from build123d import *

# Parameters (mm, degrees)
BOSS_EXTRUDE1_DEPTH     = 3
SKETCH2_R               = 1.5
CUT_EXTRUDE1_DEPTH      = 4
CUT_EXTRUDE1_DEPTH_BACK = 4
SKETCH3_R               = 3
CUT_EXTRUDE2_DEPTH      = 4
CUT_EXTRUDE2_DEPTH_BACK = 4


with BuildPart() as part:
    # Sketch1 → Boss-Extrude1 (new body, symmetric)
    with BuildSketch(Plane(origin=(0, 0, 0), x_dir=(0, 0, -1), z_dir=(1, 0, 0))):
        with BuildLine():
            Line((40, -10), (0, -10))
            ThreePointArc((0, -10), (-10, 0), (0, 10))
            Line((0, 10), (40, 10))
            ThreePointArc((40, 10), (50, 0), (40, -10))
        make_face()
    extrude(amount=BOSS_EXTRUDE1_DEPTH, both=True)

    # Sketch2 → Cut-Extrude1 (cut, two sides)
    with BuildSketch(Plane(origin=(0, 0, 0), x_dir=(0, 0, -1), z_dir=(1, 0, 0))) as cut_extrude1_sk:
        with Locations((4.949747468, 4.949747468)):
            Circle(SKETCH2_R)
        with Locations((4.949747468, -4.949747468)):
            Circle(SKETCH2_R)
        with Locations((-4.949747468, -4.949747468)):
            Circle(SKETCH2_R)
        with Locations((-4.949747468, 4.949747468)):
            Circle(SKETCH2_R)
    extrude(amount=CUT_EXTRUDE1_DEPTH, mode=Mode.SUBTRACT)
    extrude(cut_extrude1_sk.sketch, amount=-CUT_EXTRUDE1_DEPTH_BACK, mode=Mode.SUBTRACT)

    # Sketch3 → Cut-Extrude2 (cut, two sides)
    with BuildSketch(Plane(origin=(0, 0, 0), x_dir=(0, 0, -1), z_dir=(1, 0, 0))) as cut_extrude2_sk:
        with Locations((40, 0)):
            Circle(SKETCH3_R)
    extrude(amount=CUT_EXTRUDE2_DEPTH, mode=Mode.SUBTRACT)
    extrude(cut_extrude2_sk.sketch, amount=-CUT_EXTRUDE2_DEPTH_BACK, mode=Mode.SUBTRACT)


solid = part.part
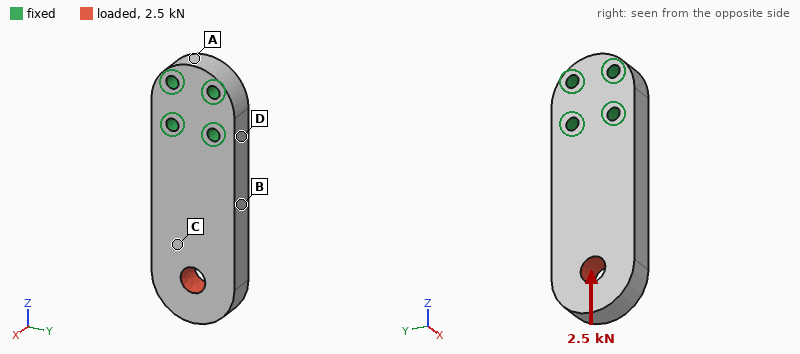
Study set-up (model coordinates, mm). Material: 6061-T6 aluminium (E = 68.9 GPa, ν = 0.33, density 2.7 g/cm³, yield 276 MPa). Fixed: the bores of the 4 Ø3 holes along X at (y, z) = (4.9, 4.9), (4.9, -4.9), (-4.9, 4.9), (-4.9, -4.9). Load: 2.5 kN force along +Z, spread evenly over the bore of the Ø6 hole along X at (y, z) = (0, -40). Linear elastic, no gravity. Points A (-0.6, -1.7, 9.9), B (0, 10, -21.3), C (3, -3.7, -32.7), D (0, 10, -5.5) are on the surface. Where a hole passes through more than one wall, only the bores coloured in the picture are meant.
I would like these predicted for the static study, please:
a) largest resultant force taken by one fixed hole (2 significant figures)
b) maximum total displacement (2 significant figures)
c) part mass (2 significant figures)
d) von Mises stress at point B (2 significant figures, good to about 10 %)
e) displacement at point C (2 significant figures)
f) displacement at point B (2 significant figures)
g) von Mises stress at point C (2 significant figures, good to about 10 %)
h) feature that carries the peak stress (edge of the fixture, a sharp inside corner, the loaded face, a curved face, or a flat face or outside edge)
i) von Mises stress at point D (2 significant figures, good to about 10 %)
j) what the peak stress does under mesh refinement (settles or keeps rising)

1.1 kN
14 µm
17 g
21 MPa
8.6 µm
5.2 µm
25 MPa
edge of the fixture
13 MPa
keeps rising
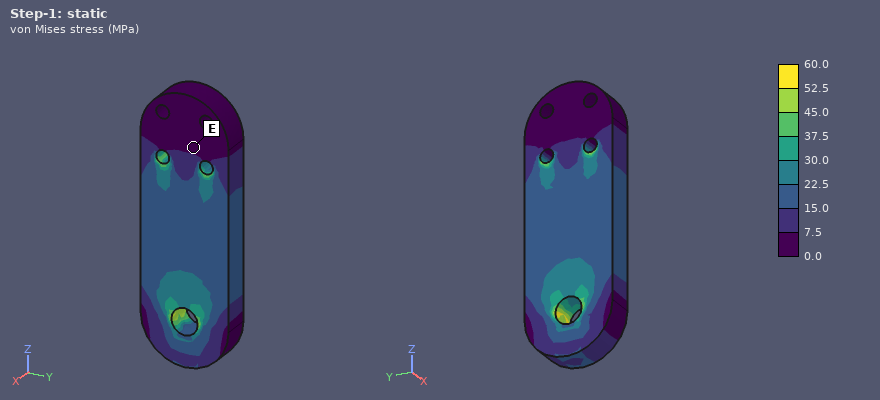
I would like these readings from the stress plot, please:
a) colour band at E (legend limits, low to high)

0.0 to 7.5 MPa
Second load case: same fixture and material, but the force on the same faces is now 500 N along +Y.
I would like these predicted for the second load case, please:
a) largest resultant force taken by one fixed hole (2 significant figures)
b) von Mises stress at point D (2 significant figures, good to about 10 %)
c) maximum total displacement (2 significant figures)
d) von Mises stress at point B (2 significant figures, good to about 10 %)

1.2 kN
29 MPa
48 µm
23 MPa
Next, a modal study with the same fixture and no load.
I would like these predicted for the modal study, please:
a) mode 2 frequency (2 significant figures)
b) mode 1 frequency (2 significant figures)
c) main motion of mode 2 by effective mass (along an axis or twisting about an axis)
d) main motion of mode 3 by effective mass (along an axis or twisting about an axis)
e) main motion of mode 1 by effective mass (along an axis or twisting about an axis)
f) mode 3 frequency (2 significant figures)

7500 Hz
2800 Hz
along Y
twisting about Z
along X
11 kHz
